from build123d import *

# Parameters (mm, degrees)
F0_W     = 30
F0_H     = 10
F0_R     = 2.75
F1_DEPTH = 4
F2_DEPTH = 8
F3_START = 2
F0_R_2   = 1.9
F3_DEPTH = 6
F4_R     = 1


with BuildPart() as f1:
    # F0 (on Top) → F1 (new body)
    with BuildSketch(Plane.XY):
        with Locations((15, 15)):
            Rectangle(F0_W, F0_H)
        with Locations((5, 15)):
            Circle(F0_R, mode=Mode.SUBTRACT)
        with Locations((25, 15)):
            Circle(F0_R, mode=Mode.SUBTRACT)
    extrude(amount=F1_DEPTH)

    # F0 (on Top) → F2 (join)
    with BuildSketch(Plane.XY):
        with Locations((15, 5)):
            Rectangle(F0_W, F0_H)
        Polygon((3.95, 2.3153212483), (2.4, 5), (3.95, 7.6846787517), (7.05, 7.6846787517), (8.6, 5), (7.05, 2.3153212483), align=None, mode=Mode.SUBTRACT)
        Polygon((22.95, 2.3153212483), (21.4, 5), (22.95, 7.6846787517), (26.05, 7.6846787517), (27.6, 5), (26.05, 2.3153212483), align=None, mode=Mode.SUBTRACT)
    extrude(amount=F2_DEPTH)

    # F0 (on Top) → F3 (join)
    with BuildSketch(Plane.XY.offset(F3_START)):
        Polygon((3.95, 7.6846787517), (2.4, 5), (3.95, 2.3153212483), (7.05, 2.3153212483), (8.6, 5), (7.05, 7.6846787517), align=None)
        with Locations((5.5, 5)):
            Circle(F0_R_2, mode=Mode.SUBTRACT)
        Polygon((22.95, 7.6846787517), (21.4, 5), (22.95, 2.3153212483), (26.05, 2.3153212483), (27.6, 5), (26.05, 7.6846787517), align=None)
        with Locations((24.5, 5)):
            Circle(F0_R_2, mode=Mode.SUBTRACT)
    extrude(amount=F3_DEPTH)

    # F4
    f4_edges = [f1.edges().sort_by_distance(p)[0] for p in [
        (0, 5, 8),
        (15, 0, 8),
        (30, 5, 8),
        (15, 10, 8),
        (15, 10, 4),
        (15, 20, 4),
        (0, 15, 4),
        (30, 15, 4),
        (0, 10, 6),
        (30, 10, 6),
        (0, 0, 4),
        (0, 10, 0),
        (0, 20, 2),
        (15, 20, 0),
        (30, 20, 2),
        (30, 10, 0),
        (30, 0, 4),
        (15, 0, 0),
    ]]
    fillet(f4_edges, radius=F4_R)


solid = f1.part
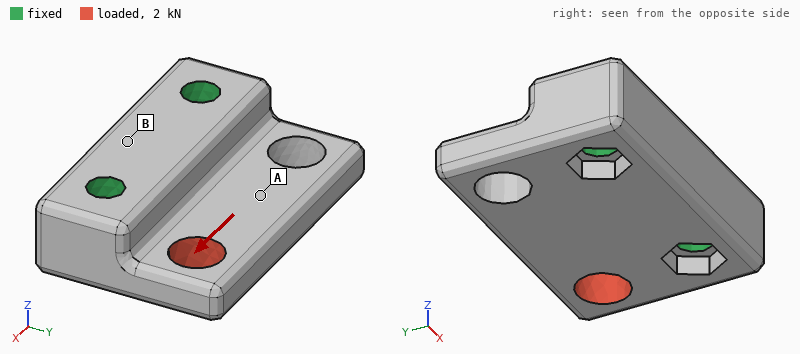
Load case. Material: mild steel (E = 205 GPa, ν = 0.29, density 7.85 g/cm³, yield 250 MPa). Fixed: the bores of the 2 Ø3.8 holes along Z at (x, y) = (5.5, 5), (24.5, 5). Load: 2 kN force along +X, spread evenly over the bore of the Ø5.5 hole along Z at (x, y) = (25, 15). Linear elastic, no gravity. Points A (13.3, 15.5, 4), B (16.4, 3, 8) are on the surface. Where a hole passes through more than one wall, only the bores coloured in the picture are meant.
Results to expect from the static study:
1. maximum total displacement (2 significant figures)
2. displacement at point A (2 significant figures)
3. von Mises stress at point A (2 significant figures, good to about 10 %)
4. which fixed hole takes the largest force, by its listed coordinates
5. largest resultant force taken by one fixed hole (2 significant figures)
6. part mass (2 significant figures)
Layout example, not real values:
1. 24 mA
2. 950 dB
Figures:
1. 7.1 µm
2. 2.5 µm
3. 32 MPa
4. (24.5, 5)
5. 1.4 kN
6. 25 g
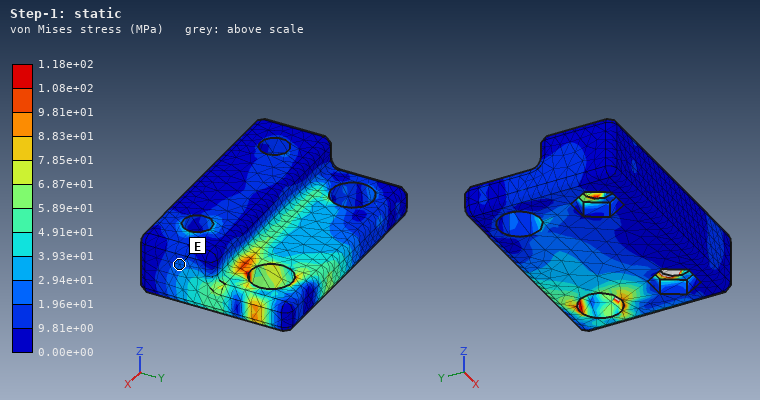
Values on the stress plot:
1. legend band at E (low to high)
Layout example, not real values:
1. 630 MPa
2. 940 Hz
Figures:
1. 1.96e+01 to 2.94e+01 MPa
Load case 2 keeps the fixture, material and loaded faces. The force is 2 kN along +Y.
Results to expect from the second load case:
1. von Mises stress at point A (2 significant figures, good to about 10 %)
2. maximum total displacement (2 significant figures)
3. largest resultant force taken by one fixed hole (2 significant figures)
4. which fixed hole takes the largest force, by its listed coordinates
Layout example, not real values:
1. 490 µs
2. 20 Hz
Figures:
1. 12 MPa
2. 7.8 µm
3. 1.9 kN
4. (24.5, 5)
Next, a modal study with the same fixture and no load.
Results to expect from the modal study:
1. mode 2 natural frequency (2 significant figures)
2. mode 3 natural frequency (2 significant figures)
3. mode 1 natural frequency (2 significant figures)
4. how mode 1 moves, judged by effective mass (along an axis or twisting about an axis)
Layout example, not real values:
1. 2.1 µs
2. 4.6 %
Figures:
1. 26 kHz
2. 39 kHz
3. 19 kHz
4. along Z
